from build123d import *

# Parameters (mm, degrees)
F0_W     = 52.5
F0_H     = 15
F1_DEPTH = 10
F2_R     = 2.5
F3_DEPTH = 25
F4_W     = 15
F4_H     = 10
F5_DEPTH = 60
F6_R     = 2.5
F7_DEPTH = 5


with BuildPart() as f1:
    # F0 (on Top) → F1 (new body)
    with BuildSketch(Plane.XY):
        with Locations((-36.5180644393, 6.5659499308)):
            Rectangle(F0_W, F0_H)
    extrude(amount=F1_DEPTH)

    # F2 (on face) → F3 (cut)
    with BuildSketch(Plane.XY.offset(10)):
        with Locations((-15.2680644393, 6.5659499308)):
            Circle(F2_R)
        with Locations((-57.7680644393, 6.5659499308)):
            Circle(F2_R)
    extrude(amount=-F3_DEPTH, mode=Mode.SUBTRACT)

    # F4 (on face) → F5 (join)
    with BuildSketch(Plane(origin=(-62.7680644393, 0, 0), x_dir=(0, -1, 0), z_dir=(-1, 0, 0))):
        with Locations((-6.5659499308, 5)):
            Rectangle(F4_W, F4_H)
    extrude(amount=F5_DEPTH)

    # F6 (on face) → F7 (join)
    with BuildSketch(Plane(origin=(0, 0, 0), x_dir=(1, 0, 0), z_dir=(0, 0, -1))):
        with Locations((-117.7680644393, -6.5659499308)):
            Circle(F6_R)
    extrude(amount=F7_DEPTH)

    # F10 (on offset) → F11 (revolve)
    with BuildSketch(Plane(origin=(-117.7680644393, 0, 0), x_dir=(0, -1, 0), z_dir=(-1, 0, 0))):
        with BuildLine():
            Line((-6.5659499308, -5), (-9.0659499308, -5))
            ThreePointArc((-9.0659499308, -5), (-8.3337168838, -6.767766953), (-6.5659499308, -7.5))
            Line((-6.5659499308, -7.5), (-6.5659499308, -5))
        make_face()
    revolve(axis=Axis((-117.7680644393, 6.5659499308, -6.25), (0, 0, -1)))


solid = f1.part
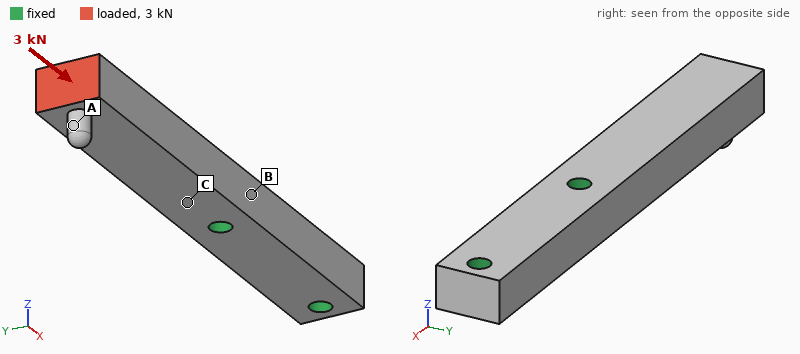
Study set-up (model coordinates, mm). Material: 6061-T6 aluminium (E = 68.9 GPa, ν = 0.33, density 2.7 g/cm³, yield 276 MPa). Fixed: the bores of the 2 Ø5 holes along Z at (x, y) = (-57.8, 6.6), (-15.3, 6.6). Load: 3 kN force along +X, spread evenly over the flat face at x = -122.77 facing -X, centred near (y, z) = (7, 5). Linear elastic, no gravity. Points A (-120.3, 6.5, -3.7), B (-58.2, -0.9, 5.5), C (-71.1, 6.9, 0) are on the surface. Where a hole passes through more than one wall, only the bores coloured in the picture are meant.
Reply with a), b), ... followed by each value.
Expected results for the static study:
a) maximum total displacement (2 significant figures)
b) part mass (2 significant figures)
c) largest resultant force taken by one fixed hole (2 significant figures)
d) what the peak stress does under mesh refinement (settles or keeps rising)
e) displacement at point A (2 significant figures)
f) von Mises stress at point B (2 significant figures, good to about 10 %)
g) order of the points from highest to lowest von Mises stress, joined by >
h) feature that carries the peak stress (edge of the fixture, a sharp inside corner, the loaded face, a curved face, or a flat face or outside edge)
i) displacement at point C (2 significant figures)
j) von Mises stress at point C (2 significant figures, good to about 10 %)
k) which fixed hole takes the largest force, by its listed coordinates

a) 19 µm
b) 45 g
c) 2.9 kN
d) keeps rising
e) 18 µm
f) 10 MPa
g) C > B > A
h) edge of the fixture
i) 4.1 µm
j) 21 MPa
k) (-57.8, 6.6)
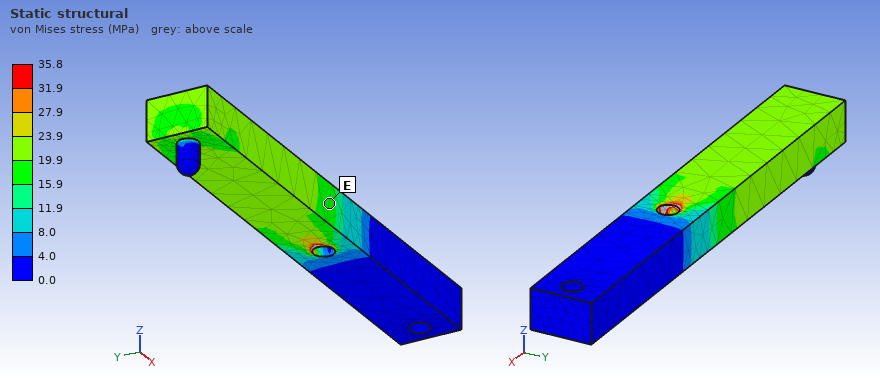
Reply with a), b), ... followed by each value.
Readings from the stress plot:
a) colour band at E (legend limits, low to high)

a) 15.9 to 19.9 MPa
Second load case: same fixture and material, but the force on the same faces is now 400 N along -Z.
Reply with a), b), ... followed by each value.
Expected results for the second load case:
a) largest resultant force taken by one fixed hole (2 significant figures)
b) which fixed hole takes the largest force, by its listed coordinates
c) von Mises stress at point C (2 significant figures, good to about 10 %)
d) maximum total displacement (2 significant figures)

a) 460 N
b) (-57.8, 6.6)
c) 83 MPa
d) 0.43 mm
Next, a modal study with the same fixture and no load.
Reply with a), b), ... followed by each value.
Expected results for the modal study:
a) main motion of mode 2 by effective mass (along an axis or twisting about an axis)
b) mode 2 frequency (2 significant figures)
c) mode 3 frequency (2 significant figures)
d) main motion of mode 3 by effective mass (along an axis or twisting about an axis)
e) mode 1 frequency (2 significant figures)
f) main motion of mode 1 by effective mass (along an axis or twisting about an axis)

a) along Y
b) 2400 Hz
c) 9900 Hz
d) twisting about X
e) 1900 Hz
f) along Z
